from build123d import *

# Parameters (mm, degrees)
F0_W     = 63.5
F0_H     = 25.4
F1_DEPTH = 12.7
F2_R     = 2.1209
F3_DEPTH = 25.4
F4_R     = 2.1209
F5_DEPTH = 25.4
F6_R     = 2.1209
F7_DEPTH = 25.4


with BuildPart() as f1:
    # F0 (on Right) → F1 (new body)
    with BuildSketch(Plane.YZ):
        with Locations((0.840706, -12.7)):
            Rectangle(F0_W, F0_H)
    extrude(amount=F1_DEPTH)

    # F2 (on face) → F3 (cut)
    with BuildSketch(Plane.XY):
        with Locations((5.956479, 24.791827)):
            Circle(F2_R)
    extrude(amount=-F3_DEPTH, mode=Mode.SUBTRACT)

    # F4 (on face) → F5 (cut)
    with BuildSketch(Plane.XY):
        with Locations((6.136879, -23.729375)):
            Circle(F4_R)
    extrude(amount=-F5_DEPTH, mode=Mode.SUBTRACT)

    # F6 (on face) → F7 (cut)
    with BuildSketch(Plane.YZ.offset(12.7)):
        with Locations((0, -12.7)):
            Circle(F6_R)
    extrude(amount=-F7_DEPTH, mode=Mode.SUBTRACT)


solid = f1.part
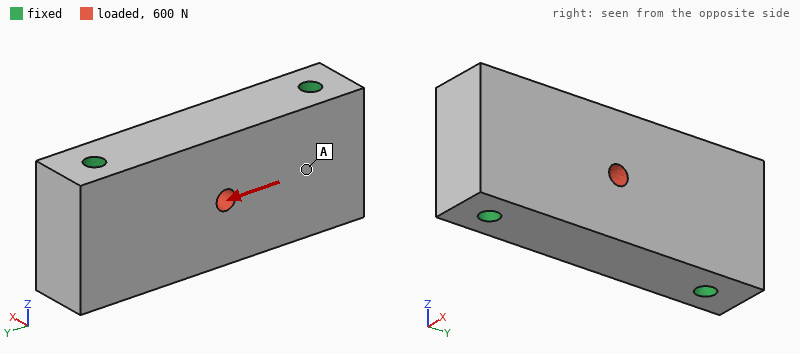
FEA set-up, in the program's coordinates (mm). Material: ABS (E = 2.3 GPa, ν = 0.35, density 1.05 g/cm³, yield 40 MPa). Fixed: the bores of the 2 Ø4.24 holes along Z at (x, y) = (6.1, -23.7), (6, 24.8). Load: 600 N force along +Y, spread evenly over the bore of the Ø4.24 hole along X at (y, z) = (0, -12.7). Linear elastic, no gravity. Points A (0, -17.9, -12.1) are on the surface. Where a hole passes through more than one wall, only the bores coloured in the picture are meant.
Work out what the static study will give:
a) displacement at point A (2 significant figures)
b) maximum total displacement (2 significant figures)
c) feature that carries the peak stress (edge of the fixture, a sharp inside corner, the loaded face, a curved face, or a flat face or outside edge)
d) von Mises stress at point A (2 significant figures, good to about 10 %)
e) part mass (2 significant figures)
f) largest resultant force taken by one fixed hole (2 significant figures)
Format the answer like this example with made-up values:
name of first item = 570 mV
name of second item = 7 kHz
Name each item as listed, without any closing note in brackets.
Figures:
displacement at point A = 3.2 µm
maximum total displacement = 16 µm
feature that carries the peak stress = the loaded face
von Mises stress at point A = 0.85 MPa
part mass = 21 g
largest resultant force taken by one fixed hole = 310 N
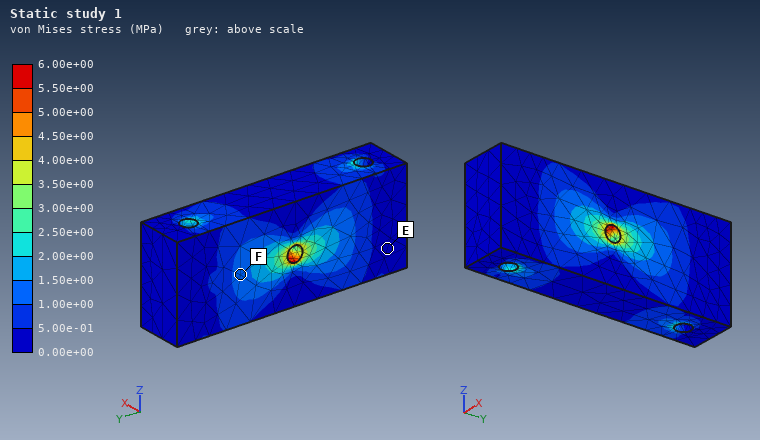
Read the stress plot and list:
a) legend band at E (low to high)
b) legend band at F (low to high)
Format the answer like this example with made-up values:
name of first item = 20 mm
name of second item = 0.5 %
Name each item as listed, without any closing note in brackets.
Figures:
legend band at E = 0.00e+00 to 5.00e-01 MPa
legend band at F = 1.00e+00 to 1.50e+00 MPa
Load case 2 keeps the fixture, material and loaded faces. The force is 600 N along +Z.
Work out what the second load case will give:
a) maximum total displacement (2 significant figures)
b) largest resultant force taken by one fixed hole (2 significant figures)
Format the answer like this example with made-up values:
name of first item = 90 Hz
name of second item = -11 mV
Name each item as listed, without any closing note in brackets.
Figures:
maximum total displacement = 41 µm
largest resultant force taken by one fixed hole = 310 N
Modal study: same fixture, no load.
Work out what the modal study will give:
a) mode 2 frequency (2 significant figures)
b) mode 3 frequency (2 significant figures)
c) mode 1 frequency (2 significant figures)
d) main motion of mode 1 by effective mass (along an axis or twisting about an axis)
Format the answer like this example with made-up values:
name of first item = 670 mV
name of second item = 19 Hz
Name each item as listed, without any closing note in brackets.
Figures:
mode 2 frequency = 7600 Hz
mode 3 frequency = 7900 Hz
mode 1 frequency = 5100 Hz
main motion of mode 1 by effective mass = along X
